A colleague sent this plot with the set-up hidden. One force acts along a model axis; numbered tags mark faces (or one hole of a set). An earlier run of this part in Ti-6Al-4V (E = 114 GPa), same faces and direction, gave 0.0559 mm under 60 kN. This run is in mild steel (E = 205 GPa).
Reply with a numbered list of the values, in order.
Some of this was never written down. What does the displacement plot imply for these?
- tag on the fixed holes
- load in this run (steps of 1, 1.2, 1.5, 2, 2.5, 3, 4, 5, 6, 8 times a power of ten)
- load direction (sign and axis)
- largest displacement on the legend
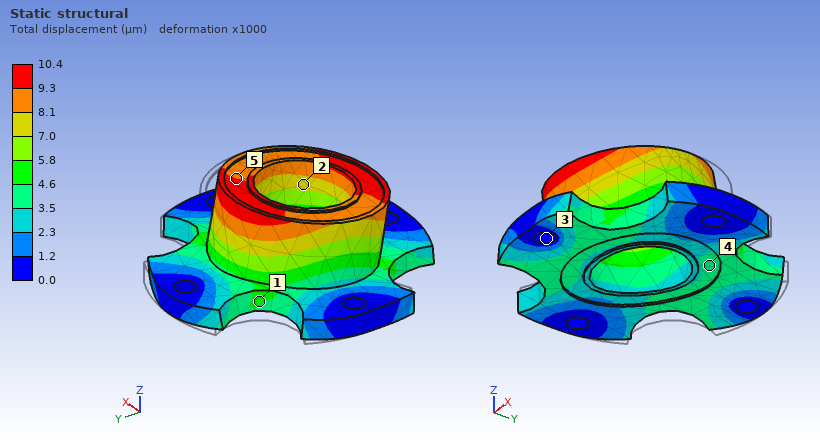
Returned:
1. 3
2. 20 kN
3. -Y
4. 10.4 µm
